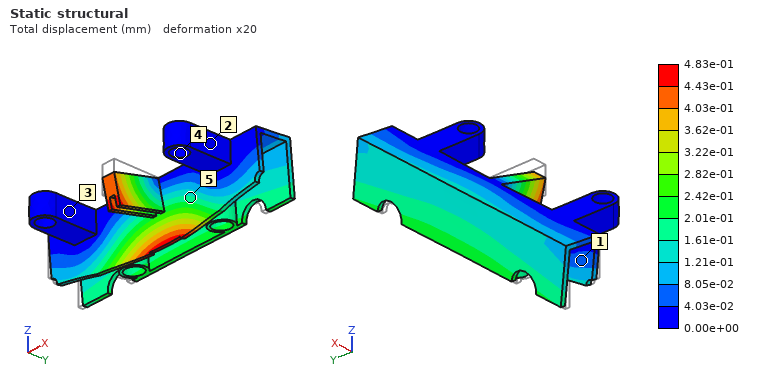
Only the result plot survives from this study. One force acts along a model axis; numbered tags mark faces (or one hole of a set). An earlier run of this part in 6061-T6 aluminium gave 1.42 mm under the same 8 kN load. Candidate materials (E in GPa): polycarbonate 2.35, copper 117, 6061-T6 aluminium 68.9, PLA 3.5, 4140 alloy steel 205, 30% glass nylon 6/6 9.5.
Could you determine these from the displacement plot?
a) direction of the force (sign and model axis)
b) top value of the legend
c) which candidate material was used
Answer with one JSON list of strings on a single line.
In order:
["+Y", "4.83e-01 mm", "4140 alloy steel"]
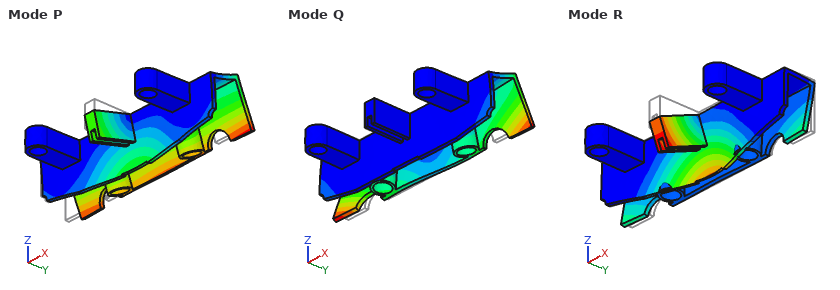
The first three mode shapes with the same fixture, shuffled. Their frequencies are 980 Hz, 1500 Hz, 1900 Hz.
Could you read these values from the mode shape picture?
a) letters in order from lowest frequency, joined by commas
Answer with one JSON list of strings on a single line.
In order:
["P, Q, R"]
